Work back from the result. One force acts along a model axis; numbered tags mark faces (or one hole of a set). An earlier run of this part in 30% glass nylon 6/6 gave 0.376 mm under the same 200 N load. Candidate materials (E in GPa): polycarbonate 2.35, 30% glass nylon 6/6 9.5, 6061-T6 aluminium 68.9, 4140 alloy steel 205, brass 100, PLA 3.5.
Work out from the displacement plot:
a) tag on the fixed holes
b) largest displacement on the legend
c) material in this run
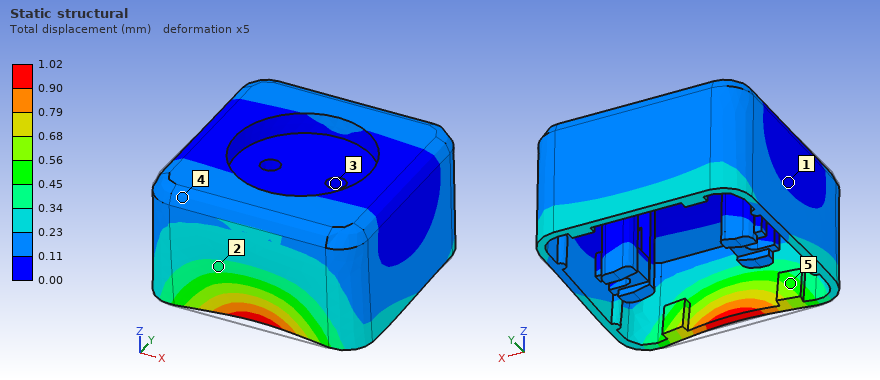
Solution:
3
1.02 mm
PLA
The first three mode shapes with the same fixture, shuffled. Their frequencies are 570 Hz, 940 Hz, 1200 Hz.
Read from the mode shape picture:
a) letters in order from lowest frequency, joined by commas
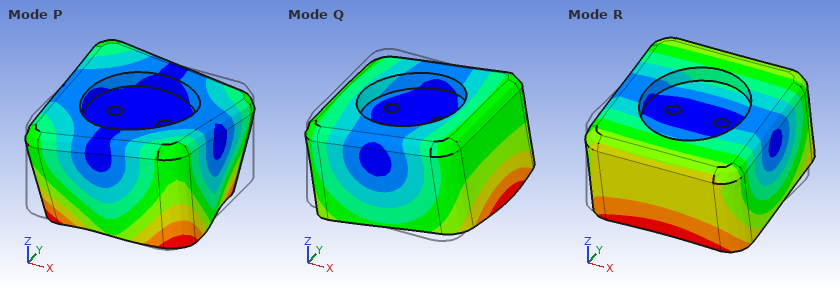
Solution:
R, Q, P
